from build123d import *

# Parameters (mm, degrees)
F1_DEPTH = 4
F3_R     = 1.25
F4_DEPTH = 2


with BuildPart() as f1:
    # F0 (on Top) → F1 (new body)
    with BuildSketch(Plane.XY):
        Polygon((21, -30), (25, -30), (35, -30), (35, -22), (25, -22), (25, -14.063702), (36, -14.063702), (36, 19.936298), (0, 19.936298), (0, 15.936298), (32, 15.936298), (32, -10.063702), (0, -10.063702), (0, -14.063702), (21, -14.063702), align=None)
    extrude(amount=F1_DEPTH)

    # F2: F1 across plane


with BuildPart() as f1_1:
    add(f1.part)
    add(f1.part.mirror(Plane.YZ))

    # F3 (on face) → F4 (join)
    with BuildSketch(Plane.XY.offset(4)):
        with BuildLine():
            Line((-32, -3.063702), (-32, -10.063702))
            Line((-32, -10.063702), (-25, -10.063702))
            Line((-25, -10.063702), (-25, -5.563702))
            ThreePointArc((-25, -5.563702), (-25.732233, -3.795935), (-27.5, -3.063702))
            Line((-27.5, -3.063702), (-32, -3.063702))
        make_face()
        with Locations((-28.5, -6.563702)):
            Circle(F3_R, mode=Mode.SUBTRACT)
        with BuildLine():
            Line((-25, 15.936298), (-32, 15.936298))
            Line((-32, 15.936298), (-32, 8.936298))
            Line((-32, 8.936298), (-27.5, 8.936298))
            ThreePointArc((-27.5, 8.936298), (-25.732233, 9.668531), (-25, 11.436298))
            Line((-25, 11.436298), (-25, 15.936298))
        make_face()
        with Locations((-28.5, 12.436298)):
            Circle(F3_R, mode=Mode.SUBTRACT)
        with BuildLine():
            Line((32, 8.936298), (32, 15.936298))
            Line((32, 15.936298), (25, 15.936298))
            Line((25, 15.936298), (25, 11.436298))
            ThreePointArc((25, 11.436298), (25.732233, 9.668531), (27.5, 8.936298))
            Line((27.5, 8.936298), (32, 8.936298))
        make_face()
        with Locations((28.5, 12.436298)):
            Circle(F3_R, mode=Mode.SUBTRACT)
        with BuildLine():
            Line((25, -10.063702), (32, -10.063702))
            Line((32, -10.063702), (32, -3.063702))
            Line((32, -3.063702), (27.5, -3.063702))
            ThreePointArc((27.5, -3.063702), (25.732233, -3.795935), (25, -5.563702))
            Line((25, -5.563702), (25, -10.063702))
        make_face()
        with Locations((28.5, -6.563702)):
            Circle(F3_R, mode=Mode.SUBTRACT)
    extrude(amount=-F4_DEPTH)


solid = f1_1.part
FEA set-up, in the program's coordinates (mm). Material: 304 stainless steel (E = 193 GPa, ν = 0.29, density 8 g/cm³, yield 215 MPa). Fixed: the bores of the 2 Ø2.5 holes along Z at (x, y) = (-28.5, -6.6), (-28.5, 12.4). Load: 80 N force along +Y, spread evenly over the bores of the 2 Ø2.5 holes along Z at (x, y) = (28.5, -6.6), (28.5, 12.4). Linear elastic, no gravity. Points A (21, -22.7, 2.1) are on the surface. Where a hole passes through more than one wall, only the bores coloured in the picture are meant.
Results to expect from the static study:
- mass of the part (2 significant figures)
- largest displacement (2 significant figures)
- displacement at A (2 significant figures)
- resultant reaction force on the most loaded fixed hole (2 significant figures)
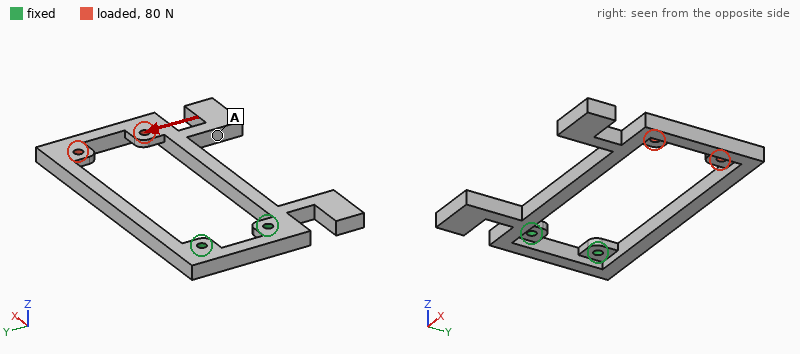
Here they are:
37 g
0.19 mm
0.16 mm
140 N
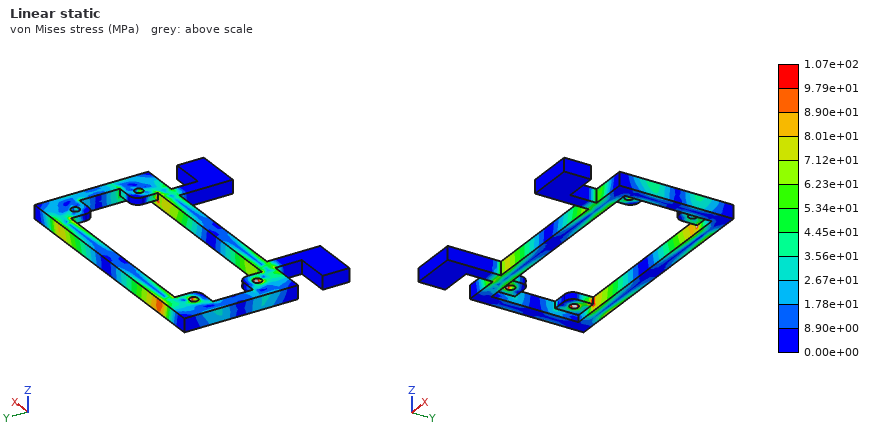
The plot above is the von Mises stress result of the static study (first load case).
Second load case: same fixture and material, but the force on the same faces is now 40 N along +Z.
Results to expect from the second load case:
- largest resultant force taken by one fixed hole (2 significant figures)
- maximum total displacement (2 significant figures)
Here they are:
21 N
0.46 mm
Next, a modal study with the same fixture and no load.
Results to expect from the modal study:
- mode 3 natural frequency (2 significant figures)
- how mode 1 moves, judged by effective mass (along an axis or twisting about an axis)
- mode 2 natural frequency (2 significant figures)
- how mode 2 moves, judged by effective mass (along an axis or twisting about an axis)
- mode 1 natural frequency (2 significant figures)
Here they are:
940 Hz
along Z
830 Hz
along Y
390 Hz
